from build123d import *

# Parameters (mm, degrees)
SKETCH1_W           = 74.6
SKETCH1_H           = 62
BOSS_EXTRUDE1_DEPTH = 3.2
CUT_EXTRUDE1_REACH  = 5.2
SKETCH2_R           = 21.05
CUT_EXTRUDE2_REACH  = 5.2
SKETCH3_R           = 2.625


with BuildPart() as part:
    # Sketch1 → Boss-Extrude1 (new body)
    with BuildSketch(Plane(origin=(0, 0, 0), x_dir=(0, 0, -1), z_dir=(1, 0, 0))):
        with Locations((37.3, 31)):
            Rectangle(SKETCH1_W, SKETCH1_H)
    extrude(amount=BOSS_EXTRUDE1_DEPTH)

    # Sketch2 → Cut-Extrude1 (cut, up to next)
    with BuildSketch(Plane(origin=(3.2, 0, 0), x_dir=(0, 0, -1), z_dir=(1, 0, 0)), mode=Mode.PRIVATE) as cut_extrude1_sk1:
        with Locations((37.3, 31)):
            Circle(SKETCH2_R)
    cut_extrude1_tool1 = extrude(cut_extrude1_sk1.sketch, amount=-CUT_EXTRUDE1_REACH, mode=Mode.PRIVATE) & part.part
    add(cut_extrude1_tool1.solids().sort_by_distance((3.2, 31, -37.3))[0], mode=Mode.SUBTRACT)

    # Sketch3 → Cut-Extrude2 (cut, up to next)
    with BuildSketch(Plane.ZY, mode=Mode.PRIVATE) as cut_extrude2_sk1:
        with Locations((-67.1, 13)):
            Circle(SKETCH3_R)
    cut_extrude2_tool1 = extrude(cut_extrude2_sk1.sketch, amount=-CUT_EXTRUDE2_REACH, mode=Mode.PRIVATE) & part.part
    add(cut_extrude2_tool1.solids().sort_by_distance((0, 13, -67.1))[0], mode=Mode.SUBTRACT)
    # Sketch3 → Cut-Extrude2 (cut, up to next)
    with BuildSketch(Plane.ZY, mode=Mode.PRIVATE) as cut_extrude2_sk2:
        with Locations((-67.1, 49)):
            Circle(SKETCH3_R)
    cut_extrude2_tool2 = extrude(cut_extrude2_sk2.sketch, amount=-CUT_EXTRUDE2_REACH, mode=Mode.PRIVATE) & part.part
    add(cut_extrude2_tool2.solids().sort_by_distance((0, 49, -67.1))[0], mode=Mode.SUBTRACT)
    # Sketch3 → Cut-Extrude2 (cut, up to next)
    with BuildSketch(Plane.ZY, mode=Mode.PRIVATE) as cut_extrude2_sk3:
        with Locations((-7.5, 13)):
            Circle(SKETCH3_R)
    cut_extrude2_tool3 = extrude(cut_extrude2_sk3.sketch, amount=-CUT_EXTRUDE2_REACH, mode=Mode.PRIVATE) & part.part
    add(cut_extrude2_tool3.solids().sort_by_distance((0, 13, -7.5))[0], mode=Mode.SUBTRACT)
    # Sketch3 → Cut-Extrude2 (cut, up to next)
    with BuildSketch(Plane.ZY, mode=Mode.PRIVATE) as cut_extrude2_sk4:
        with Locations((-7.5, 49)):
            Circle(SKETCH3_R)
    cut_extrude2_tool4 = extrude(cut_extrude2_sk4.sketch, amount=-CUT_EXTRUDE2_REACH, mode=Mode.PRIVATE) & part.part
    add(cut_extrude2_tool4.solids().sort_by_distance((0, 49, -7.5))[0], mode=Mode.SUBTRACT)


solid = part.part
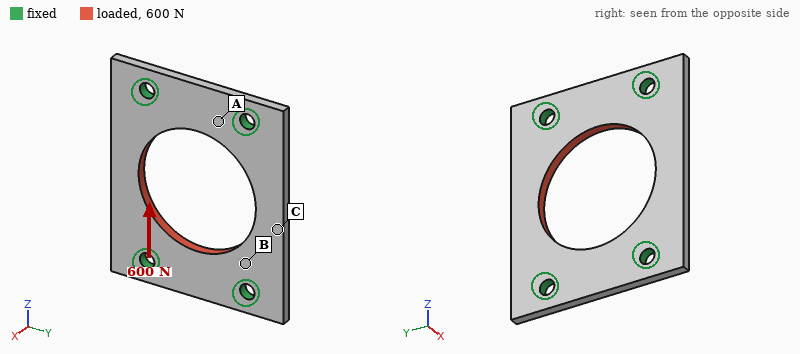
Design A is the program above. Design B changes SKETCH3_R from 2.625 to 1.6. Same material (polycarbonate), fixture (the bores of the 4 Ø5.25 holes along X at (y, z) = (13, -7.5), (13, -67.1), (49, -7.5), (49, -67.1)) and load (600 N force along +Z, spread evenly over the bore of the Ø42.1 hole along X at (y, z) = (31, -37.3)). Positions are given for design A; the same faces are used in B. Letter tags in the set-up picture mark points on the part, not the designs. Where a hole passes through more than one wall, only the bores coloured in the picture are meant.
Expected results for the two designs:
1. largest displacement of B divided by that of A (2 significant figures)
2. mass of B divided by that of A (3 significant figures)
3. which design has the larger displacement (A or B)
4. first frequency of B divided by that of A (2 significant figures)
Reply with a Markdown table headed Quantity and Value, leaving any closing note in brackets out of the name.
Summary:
| Quantity | Value |
|---|---|
| largest displacement of B divided by that of A | 1.1 |
| mass of B divided by that of A | 1.02 |
| which design has the larger displacement | B |
| first frequency of B divided by that of A | 0.90 |
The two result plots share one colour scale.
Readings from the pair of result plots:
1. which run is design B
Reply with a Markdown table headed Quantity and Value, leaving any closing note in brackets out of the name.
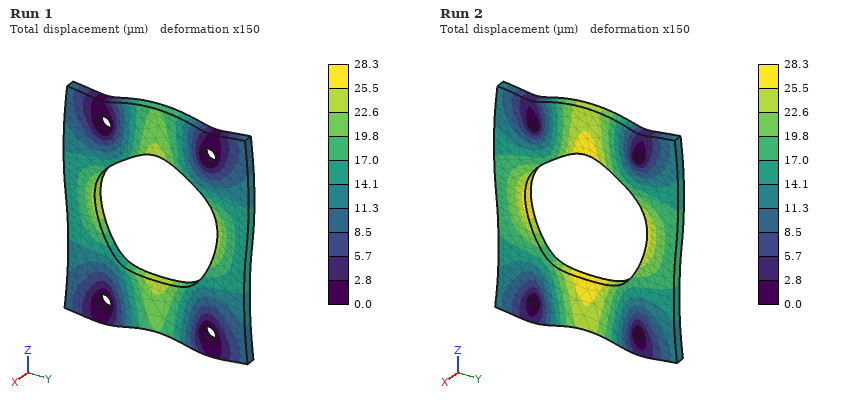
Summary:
| Quantity | Value |
|---|---|
| which run is design B | Run 2 |
